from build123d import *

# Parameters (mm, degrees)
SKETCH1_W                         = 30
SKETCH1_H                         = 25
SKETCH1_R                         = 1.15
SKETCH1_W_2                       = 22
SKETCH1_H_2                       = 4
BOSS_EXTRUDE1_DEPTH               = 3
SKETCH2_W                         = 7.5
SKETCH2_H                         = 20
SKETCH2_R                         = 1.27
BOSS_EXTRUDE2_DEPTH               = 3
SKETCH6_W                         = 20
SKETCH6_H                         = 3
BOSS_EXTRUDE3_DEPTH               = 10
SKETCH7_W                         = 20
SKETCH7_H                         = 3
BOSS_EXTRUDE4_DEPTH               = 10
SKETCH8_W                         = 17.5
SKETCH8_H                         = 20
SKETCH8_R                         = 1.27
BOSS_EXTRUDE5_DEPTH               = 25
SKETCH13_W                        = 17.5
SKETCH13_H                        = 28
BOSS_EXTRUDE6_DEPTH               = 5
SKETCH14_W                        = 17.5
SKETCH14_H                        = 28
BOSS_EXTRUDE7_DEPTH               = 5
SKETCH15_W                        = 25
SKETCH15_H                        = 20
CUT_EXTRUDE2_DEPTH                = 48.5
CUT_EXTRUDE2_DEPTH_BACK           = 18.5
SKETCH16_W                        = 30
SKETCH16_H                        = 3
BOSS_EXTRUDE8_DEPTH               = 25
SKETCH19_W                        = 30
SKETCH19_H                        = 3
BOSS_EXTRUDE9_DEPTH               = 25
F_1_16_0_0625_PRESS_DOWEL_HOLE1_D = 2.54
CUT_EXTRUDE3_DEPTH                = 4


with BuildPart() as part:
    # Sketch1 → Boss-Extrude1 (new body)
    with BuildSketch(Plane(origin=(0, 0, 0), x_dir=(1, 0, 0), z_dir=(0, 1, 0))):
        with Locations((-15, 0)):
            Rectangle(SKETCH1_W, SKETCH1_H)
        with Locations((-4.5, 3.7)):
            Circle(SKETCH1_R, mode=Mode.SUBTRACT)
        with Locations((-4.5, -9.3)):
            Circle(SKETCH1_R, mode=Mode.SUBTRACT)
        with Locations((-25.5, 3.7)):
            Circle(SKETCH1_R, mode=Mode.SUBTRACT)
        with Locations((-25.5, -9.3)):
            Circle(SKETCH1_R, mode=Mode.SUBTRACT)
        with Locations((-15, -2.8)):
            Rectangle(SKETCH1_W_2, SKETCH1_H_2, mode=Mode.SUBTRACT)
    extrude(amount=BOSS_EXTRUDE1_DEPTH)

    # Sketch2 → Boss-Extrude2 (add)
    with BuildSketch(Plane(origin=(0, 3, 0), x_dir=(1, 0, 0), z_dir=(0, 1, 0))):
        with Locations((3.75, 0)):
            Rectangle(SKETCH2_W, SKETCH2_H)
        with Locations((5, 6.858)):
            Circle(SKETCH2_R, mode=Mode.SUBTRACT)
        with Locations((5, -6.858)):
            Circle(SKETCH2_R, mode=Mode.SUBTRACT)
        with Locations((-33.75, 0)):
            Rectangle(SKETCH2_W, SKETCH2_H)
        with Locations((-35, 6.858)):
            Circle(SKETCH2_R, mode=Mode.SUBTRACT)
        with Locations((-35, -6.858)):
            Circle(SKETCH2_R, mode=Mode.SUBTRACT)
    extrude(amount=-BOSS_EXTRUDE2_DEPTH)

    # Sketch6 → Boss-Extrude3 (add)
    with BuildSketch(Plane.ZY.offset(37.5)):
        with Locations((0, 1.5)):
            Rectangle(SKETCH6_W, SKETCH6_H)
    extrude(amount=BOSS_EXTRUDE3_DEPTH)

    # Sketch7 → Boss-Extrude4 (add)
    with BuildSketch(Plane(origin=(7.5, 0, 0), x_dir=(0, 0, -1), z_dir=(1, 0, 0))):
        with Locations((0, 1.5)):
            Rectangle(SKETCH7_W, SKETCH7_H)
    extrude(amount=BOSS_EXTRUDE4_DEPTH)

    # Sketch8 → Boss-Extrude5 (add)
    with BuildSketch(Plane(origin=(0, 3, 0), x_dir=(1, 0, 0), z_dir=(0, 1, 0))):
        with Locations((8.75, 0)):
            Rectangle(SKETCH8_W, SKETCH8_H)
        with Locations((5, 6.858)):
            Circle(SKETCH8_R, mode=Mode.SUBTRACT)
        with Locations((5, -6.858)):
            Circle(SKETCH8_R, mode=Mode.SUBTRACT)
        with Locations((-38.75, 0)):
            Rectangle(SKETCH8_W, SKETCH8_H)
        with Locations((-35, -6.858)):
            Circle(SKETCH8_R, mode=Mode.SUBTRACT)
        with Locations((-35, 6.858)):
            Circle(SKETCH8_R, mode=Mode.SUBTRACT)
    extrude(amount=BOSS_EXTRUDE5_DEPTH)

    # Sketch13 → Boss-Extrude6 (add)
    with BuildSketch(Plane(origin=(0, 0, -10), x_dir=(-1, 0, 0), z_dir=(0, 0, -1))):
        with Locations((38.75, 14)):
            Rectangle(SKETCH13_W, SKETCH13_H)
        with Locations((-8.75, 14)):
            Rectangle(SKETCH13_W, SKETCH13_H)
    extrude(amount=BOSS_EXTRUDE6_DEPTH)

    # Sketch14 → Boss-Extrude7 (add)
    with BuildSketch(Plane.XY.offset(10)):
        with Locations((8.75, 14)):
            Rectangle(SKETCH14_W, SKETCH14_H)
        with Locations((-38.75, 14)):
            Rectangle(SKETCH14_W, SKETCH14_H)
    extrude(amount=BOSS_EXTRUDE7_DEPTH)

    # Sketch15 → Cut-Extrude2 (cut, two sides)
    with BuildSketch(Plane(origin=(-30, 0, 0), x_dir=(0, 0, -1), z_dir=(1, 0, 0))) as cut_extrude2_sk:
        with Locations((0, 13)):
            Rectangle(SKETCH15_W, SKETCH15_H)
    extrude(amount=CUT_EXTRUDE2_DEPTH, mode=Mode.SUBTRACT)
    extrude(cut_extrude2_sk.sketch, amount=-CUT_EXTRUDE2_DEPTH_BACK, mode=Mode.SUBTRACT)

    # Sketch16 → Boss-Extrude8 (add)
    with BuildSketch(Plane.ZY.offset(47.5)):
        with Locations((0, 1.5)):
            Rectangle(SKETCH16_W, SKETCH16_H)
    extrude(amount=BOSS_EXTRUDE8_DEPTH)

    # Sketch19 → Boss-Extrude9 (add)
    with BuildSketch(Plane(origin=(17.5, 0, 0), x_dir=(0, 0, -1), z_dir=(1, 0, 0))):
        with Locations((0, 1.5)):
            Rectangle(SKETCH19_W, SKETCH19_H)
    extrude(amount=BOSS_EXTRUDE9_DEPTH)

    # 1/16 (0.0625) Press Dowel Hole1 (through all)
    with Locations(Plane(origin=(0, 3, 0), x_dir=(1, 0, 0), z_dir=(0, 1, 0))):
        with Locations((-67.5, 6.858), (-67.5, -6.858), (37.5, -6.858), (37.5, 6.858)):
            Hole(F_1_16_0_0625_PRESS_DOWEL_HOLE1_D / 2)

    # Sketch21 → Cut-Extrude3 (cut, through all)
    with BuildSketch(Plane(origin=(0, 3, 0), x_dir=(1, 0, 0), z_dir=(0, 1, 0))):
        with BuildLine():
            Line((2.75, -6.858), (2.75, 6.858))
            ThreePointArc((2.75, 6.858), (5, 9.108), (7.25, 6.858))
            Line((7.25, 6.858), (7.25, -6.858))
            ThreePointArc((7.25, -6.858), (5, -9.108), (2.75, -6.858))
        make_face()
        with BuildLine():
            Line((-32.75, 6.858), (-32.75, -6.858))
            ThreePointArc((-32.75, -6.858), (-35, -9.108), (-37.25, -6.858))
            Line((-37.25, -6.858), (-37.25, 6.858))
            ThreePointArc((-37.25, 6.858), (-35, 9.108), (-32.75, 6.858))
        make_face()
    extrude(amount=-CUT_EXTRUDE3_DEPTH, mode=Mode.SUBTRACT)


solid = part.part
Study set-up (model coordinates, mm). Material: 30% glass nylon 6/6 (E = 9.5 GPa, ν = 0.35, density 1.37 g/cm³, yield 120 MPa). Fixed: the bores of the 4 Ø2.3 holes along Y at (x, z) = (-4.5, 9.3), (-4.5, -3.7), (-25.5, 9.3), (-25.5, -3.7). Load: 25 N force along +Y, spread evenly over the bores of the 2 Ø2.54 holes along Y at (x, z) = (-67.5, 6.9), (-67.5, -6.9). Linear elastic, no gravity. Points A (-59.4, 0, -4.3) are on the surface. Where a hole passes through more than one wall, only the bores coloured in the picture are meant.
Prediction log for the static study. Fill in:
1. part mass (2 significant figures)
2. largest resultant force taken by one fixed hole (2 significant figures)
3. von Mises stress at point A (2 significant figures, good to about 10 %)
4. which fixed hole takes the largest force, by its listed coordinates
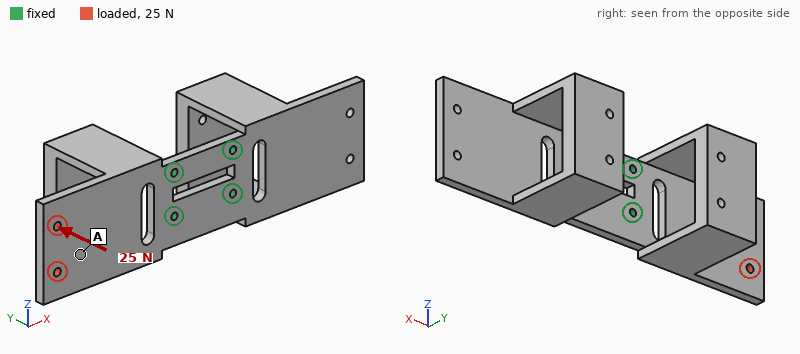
24 g
26 N
5.4 MPa
(-25.5, -3.7)
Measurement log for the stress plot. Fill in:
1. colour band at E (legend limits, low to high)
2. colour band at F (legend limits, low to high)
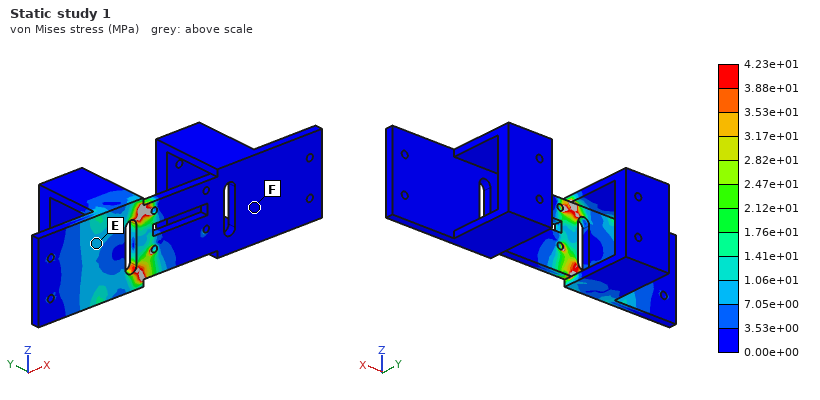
7.05e+00 to 1.06e+01 MPa
0.00e+00 to 3.53e+00 MPa
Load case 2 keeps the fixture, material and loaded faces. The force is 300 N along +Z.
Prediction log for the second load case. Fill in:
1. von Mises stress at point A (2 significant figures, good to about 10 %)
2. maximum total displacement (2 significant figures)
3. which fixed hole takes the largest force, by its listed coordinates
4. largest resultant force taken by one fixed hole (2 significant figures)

8.0 MPa
0.47 mm
(-25.5, 9.3)
650 N
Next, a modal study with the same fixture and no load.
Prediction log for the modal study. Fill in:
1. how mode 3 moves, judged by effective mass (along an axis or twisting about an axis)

along Z
